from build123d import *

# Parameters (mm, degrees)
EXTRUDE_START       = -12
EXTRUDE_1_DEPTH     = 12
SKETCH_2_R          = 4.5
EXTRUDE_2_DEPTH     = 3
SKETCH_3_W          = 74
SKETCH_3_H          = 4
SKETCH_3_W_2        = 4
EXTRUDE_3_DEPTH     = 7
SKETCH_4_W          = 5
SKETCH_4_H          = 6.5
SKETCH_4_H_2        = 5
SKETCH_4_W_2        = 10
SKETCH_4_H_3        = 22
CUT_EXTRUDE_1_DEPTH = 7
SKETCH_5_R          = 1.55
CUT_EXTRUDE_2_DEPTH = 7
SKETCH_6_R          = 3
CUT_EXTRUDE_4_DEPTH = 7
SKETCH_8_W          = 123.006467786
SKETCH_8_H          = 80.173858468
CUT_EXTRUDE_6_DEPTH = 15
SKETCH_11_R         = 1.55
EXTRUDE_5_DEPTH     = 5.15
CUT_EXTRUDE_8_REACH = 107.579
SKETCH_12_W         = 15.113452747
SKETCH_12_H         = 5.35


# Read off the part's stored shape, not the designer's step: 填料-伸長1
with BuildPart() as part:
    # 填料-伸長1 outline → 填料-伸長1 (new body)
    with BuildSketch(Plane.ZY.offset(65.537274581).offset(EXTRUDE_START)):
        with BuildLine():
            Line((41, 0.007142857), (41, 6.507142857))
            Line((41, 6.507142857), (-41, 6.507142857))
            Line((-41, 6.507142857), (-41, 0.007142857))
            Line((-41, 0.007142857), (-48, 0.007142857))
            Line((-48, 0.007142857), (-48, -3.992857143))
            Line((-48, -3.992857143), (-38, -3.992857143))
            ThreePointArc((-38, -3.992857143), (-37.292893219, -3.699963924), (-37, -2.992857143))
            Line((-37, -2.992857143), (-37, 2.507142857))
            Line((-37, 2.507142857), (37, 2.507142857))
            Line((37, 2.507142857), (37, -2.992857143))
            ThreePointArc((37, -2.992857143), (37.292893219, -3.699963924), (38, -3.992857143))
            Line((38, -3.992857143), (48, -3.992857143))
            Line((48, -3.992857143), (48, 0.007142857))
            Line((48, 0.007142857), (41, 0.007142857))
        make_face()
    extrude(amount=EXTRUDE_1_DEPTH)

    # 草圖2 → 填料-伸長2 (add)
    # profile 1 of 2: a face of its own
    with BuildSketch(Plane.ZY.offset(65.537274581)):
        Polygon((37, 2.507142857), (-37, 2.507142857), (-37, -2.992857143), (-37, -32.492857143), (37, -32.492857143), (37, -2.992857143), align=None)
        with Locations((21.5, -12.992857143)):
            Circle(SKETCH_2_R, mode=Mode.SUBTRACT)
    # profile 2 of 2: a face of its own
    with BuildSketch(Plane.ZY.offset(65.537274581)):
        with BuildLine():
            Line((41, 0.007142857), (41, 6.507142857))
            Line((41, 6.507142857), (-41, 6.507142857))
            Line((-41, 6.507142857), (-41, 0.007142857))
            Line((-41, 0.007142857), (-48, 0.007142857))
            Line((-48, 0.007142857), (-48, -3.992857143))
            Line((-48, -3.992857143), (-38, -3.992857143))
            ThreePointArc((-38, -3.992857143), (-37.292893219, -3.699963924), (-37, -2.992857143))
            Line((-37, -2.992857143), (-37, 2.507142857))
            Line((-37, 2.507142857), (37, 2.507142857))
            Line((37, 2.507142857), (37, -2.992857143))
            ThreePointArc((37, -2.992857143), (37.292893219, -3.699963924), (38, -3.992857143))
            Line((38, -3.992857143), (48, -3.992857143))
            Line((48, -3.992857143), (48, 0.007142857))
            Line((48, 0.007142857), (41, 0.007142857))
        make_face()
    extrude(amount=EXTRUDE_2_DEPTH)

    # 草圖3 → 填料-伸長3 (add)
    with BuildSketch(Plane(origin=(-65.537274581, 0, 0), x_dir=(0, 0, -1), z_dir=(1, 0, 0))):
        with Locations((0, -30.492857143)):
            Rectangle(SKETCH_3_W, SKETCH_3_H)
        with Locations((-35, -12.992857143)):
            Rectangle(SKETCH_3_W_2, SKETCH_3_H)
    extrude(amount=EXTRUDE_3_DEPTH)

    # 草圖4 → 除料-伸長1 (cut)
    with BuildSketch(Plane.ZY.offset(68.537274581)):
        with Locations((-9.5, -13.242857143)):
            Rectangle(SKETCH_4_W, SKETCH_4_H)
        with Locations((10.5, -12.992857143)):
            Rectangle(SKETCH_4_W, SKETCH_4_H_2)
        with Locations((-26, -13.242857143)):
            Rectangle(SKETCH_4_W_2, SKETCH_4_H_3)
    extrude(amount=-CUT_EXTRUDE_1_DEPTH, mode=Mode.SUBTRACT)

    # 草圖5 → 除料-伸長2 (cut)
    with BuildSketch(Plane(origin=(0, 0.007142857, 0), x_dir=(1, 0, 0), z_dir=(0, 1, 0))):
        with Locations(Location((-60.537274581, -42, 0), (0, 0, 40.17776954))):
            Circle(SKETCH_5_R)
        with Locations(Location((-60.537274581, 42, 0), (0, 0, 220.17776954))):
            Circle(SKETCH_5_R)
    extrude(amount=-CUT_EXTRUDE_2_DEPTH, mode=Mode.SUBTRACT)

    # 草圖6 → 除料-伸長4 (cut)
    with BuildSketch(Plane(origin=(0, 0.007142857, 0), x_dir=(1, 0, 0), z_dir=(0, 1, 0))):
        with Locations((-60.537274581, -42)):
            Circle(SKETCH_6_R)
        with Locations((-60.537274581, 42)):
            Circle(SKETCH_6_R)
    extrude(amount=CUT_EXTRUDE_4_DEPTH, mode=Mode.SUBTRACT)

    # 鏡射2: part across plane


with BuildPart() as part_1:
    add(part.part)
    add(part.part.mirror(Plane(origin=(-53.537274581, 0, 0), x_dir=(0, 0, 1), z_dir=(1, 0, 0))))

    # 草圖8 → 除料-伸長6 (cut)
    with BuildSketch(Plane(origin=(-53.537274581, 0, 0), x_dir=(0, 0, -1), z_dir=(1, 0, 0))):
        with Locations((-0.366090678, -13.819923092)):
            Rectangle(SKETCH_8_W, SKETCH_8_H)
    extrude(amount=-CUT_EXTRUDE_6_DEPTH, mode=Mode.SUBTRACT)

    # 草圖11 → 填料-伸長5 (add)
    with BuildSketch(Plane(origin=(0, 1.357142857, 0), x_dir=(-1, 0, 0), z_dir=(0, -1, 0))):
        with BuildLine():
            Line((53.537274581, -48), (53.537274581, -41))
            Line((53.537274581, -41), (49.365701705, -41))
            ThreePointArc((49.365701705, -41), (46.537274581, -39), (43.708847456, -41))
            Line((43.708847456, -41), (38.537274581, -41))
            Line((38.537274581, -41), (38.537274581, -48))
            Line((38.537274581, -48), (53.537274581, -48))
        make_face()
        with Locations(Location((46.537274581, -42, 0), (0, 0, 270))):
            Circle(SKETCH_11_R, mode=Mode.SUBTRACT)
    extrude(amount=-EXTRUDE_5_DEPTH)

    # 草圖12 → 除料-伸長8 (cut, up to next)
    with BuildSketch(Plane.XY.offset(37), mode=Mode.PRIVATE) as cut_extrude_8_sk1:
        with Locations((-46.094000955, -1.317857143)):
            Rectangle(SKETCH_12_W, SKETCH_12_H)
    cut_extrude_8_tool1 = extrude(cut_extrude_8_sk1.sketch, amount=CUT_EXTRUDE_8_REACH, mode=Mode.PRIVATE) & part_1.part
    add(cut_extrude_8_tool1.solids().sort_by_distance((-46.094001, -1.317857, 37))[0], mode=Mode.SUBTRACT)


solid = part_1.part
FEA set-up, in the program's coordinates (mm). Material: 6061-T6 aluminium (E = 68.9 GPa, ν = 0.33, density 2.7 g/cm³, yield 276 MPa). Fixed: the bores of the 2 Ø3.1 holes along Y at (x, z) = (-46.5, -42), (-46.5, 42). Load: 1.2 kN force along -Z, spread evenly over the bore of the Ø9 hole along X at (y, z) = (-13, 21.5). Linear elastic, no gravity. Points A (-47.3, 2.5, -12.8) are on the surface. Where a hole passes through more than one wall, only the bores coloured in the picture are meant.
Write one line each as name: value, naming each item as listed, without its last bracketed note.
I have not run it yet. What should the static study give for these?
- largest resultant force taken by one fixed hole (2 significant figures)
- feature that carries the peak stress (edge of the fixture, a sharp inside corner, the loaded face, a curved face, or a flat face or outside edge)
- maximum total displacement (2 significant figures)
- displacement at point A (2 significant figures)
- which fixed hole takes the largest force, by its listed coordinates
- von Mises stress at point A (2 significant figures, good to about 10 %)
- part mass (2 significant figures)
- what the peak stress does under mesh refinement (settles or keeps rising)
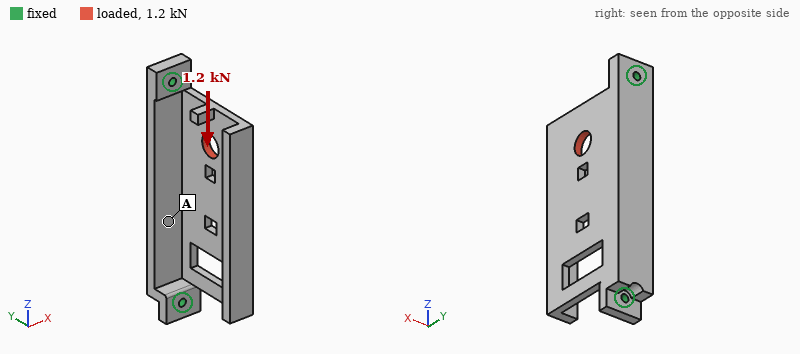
largest resultant force taken by one fixed hole: 980 N
feature that carries the peak stress: edge of the fixture
maximum total displacement: 40 µm
displacement at point A: 17 µm
which fixed hole takes the largest force, by its listed coordinates: (-46.5, 42)
von Mises stress at point A: 8.3 MPa
part mass: 41 g
what the peak stress does under mesh refinement: keeps rising
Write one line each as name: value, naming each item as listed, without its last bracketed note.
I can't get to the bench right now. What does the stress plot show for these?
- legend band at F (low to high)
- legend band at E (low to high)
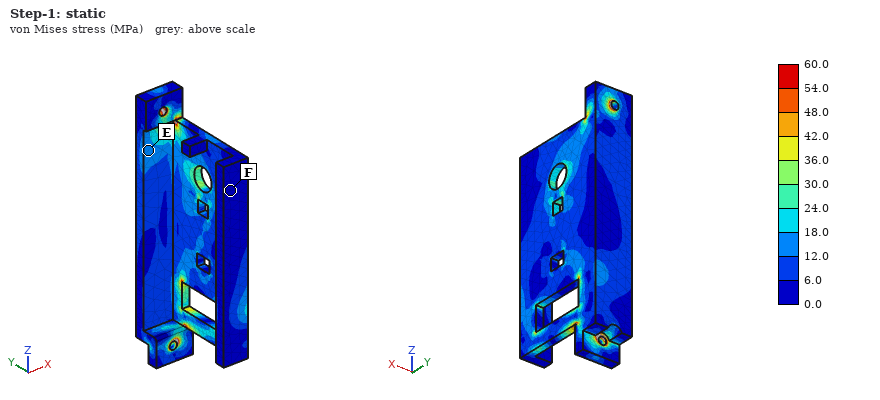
legend band at F: 0.0 to 6.0 MPa
legend band at E: 12.0 to 18.0 MPa
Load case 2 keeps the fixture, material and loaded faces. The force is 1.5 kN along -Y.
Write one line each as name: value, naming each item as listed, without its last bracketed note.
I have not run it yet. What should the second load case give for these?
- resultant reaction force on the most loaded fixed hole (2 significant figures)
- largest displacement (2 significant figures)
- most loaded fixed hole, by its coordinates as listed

resultant reaction force on the most loaded fixed hole: 1.2 kN
largest displacement: 0.16 mm
most loaded fixed hole, by its coordinates as listed: (-46.5, 42)
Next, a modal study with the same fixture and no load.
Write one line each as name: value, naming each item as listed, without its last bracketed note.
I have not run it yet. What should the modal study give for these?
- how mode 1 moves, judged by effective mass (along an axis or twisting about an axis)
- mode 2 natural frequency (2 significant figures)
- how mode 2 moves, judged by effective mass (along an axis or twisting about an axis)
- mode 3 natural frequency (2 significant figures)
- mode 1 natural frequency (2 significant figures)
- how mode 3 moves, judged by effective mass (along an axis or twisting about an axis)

how mode 1 moves, judged by effective mass: along X
mode 2 natural frequency: 2100 Hz
how mode 2 moves, judged by effective mass: twisting about Y
mode 3 natural frequency: 4300 Hz
mode 1 natural frequency: 960 Hz
how mode 3 moves, judged by effective mass: along Y
